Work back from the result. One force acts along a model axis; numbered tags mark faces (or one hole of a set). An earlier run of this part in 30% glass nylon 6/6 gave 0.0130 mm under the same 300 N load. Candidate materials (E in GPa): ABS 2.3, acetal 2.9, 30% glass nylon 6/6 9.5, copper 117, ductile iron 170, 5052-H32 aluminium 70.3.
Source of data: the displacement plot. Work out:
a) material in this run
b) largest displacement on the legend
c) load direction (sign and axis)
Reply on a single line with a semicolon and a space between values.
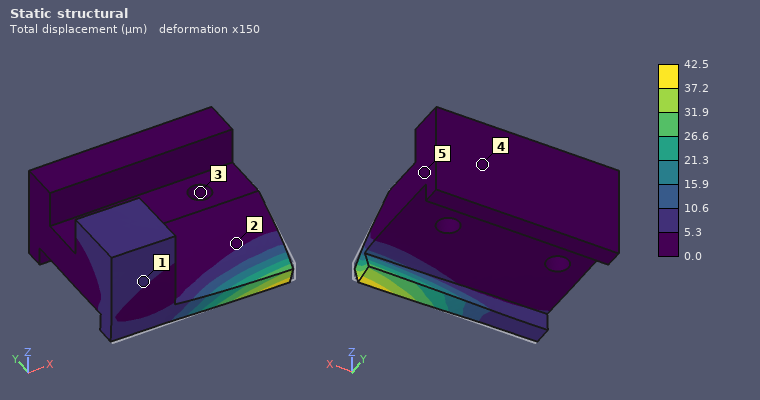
acetal; 42.5 µm; +Y
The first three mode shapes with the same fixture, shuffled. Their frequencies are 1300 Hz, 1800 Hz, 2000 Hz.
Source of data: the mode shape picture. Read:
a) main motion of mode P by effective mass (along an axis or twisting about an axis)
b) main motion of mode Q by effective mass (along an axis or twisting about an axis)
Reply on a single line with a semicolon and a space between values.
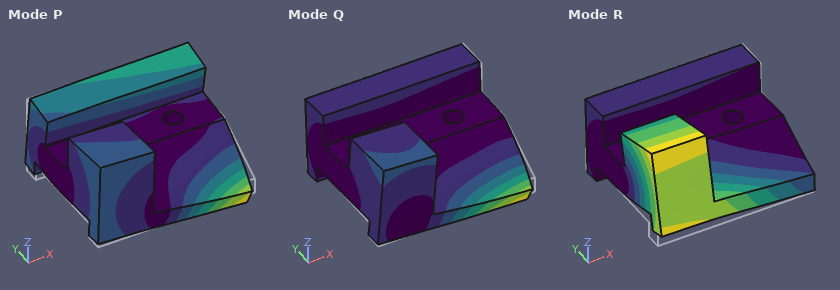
along Z; along Z
